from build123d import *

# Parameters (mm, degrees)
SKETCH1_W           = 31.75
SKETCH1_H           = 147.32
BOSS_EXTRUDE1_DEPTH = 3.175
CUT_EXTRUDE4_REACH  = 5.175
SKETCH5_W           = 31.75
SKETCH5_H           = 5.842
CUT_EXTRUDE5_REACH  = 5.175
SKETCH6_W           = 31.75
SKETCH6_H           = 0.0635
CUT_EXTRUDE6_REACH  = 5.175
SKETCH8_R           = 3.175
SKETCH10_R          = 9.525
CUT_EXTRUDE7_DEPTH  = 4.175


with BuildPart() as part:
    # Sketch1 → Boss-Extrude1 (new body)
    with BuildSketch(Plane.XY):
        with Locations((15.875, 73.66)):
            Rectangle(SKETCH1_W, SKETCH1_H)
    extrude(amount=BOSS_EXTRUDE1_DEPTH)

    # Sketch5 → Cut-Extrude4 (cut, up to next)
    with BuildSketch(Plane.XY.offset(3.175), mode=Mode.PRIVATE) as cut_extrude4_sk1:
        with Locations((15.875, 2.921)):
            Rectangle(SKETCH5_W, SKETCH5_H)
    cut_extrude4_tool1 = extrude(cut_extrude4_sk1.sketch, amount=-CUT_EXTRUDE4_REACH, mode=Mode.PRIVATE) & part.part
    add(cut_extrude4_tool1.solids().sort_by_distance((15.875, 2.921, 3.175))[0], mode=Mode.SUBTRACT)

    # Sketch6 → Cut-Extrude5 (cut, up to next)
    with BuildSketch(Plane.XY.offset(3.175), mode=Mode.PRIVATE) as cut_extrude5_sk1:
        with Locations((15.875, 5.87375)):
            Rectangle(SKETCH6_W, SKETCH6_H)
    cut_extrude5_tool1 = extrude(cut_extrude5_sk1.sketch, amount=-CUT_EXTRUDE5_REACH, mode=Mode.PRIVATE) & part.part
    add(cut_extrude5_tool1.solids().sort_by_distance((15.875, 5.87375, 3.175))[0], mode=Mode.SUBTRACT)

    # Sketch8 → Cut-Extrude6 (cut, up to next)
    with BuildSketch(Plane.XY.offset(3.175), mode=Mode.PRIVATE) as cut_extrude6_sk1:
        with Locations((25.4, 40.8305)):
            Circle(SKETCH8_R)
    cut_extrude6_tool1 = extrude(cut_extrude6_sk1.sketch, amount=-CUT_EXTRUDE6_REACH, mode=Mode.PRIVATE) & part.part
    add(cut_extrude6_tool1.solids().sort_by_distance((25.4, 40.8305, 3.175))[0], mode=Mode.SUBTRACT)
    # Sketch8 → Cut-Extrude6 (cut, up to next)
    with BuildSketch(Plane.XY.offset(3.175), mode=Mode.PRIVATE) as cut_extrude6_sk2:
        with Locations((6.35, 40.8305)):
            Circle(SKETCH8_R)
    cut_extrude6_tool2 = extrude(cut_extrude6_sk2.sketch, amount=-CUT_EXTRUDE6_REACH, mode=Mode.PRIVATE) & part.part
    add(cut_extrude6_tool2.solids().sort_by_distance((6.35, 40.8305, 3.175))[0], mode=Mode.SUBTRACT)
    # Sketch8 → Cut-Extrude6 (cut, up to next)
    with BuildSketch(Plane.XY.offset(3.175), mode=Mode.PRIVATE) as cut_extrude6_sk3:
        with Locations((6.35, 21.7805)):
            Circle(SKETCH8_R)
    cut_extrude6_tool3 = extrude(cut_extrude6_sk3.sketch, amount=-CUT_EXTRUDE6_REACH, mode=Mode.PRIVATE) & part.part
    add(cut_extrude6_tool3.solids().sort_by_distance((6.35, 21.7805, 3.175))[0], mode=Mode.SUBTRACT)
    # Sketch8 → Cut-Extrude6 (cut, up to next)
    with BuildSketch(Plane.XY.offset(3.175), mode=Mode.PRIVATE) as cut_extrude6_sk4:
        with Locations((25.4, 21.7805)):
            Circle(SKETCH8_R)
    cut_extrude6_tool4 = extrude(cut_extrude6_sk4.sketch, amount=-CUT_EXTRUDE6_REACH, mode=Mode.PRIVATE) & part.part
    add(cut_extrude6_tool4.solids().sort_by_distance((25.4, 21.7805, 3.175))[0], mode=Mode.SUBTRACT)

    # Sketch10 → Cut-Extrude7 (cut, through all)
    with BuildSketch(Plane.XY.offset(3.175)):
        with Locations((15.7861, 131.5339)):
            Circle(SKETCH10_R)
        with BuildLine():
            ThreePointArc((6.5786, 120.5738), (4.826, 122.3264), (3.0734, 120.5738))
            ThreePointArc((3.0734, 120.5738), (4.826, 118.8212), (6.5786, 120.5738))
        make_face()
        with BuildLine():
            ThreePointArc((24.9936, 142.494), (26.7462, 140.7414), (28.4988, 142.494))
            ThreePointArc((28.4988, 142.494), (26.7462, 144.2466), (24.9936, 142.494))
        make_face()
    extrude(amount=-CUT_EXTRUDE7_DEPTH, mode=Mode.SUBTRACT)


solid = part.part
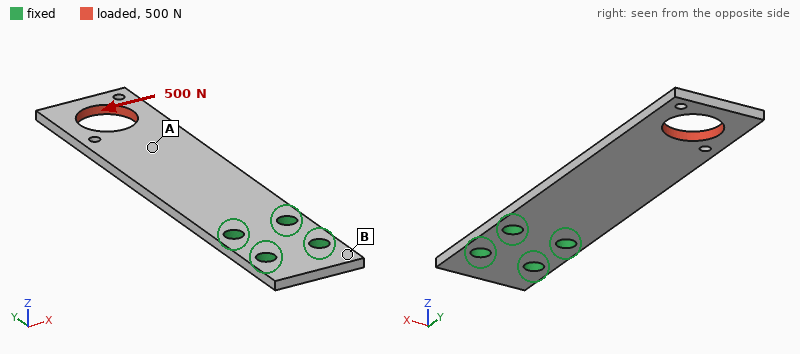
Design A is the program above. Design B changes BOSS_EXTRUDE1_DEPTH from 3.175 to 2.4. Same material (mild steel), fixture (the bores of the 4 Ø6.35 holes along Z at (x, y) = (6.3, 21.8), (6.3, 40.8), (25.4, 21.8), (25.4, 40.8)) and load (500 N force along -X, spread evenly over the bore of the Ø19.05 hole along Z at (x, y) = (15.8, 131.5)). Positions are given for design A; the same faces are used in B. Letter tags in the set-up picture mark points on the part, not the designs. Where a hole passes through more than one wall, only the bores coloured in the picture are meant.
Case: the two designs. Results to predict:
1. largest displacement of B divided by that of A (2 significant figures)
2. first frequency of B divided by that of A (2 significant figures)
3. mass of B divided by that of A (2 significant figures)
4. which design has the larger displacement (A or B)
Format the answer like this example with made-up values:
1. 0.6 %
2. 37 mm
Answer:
1. 1.3
2. 0.76
3. 0.76
4. B
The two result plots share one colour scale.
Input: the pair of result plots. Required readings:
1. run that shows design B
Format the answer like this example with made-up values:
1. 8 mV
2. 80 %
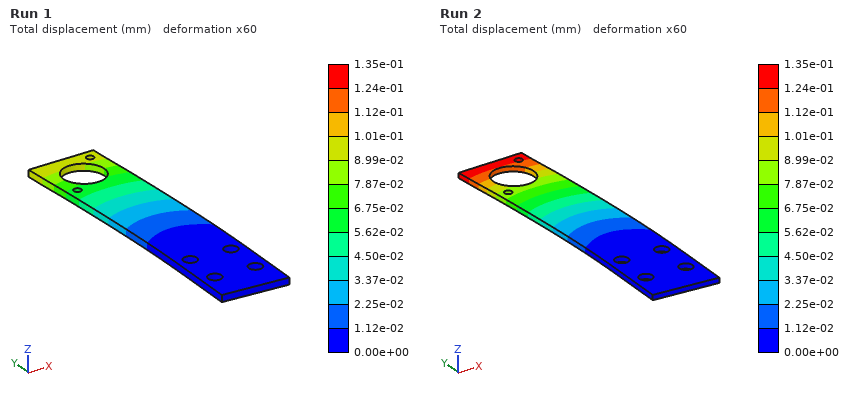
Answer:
1. Run 2
